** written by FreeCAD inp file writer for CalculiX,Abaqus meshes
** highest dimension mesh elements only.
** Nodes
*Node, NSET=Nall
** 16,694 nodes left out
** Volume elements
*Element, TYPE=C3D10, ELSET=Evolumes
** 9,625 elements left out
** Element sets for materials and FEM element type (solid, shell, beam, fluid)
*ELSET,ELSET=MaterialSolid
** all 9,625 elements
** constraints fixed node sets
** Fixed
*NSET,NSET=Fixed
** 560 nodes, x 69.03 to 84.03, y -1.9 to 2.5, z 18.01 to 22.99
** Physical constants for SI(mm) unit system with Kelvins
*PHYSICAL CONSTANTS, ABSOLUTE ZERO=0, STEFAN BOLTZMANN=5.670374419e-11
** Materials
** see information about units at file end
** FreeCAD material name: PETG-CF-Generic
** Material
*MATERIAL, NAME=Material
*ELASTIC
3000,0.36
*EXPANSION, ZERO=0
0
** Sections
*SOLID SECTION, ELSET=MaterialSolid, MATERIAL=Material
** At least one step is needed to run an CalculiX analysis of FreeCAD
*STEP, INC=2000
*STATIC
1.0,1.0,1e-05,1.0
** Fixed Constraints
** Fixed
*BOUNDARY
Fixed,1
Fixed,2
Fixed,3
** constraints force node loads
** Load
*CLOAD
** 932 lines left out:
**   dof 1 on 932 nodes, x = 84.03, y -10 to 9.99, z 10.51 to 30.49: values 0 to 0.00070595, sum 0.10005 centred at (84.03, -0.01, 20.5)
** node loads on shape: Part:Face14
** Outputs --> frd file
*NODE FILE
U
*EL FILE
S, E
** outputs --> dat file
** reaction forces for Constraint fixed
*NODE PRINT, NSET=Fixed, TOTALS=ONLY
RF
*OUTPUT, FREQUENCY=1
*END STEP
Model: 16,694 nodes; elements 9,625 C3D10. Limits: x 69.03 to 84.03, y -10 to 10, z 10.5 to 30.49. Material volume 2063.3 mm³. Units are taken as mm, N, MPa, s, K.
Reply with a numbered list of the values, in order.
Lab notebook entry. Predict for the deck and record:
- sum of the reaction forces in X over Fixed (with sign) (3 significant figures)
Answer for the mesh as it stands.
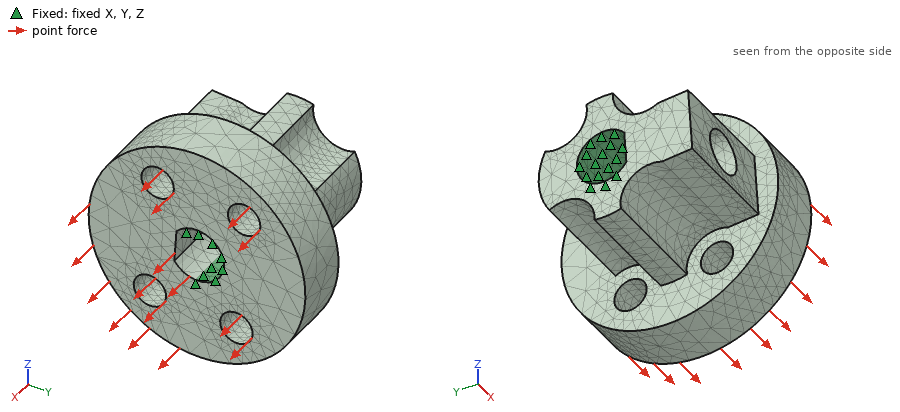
1. -0.100 N
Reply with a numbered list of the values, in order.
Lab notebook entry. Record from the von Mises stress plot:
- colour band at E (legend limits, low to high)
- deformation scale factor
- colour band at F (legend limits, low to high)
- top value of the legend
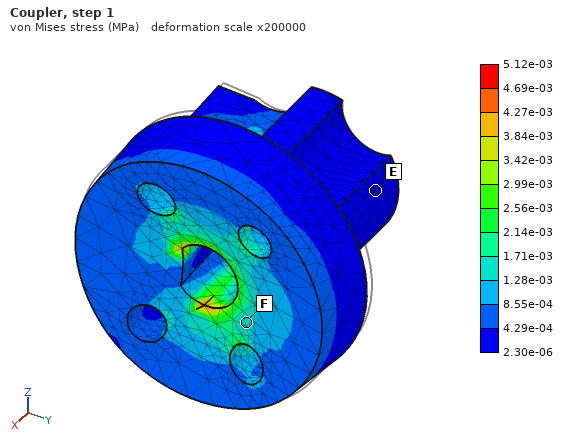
1. 2.30e-06 to 4.29e-04 MPa
2. 200000
3. 1.28e-03 to 1.71e-03 MPa
4. 5.12e-03 MPa
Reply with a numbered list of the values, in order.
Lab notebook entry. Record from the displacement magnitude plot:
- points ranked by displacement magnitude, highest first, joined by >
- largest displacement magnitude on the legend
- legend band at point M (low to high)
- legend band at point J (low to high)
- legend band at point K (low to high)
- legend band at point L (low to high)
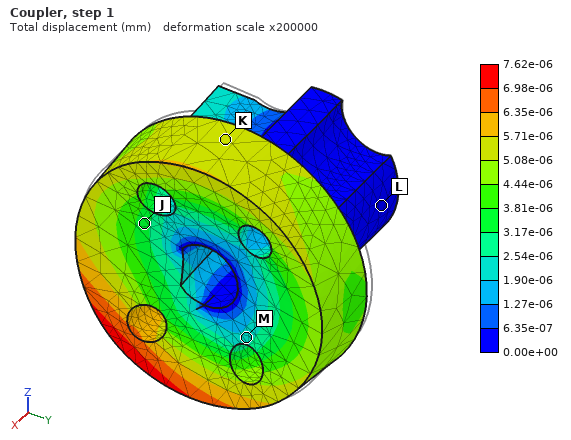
1. K > J > M > L
2. 7.62e-06 mm
3. 1.90e-06 to 2.54e-06 mm
4. 3.17e-06 to 3.81e-06 mm
5. 5.08e-06 to 5.71e-06 mm
6. 0.00e+00 to 6.35e-07 mm
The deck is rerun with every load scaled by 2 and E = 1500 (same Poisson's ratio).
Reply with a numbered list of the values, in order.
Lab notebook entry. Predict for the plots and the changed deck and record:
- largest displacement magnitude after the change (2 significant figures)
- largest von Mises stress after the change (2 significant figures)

1. 3.0e-05 mm
2. 0.010 MPa
